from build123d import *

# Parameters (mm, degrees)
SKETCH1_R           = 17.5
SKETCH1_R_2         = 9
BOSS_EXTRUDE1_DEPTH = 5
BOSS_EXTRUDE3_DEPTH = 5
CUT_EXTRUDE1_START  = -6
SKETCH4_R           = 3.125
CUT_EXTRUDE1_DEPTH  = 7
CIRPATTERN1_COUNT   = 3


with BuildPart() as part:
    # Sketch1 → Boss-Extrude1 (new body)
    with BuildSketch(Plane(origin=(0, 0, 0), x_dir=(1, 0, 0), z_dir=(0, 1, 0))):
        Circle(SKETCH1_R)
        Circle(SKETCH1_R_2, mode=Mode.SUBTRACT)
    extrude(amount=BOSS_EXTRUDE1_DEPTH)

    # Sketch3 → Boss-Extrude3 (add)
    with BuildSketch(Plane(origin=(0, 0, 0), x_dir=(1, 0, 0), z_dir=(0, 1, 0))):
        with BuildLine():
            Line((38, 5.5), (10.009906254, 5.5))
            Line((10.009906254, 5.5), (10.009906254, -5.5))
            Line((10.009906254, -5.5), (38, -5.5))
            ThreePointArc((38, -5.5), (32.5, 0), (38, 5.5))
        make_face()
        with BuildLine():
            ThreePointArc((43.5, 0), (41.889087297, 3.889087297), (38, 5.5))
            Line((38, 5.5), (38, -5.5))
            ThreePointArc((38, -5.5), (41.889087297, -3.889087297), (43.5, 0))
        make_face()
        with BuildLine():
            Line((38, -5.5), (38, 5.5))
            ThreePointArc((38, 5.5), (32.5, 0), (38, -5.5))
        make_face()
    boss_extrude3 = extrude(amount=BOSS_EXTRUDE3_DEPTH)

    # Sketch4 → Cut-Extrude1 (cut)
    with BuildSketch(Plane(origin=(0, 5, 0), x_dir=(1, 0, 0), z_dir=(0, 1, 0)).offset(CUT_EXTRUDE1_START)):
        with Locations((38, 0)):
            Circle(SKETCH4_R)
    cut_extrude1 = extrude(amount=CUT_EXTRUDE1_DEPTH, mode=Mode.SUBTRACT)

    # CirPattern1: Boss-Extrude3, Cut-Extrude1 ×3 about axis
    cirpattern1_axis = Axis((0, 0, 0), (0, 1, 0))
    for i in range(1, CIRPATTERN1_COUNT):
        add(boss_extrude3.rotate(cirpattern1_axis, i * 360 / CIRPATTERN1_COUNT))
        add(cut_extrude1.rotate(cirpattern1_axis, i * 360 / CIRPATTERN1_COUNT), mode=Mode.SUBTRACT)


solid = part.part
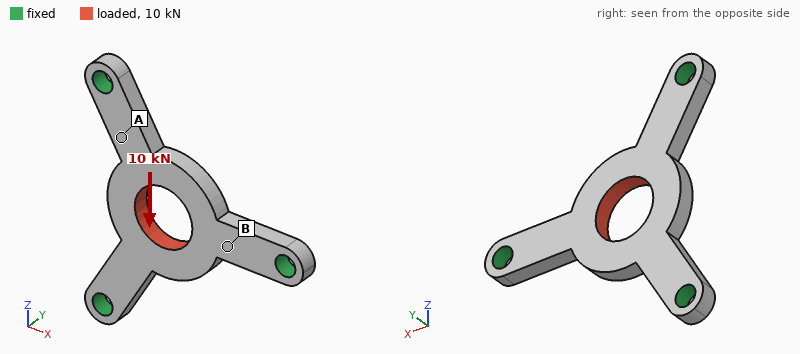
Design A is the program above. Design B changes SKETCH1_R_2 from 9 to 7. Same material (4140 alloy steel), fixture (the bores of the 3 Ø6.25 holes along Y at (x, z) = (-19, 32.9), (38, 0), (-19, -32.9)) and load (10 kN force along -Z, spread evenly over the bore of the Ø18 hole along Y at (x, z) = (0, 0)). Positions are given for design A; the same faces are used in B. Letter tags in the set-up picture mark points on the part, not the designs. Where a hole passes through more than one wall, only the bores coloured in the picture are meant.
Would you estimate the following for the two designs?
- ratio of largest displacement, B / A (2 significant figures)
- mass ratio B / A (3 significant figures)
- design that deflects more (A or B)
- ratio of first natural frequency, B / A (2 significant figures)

0.72
1.07
A
0.97
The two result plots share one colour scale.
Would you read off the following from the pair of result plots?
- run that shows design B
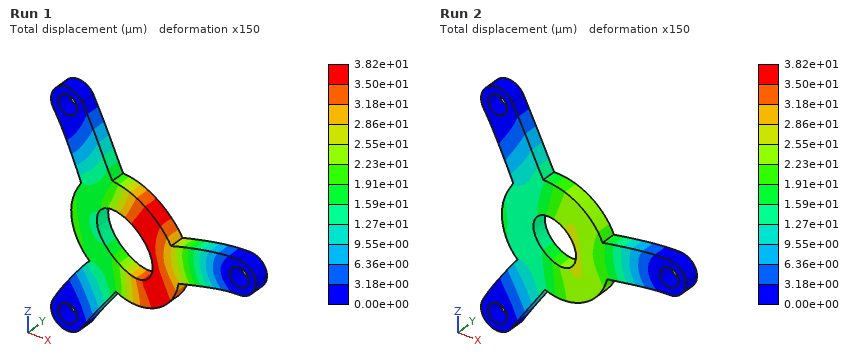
Run 2
